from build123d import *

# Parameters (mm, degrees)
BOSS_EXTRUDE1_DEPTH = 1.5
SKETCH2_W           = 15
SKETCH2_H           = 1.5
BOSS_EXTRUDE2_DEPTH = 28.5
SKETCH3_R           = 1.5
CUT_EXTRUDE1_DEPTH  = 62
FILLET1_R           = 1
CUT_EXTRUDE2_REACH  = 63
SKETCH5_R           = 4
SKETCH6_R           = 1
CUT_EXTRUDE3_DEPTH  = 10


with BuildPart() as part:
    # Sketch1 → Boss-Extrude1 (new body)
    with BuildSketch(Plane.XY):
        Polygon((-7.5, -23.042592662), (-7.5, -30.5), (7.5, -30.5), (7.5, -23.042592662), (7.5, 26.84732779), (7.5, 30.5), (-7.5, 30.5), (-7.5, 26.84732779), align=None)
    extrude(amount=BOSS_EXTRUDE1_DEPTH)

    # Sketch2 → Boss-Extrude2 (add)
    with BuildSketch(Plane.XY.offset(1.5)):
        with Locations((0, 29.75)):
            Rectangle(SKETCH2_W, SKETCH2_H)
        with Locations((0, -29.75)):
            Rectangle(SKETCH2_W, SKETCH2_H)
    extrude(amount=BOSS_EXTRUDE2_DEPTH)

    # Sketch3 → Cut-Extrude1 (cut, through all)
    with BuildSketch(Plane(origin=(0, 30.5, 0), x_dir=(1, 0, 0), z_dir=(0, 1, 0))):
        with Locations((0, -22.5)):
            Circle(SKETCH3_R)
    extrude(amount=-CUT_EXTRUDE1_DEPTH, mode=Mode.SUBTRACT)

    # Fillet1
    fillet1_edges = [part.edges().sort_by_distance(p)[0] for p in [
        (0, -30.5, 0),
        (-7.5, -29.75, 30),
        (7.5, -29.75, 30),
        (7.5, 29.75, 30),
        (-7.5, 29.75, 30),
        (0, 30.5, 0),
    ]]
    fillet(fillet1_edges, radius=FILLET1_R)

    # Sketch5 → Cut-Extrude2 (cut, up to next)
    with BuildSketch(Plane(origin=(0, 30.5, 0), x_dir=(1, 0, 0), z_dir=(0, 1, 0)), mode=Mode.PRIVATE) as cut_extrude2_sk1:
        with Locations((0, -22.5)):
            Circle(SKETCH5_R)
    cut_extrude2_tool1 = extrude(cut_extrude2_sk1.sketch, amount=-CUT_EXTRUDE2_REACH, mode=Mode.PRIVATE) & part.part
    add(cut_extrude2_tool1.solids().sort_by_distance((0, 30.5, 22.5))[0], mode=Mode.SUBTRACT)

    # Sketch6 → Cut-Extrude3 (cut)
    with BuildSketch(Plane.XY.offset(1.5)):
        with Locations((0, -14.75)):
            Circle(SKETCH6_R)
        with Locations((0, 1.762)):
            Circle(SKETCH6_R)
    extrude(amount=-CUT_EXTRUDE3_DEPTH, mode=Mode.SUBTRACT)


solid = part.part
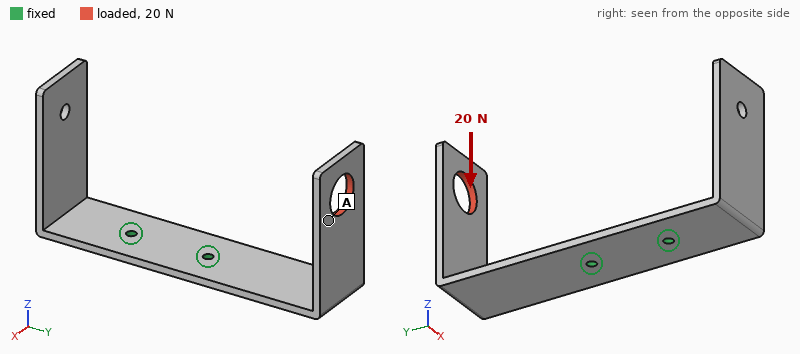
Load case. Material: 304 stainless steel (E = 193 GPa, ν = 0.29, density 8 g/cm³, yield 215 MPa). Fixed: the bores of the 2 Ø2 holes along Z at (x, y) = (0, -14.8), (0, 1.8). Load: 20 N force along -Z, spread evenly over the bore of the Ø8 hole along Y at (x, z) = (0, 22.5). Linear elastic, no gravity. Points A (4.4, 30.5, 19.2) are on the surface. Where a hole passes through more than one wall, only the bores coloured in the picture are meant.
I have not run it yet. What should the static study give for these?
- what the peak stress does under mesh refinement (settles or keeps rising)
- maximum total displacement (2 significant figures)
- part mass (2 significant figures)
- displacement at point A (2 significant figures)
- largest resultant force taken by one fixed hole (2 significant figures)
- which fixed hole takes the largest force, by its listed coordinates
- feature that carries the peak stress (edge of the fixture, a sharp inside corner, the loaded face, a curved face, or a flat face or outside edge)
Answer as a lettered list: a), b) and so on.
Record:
a) keeps rising
b) 0.34 mm
c) 20 g
d) 0.26 mm
e) 28 N
f) (0, 1.8)
g) edge of the fixture
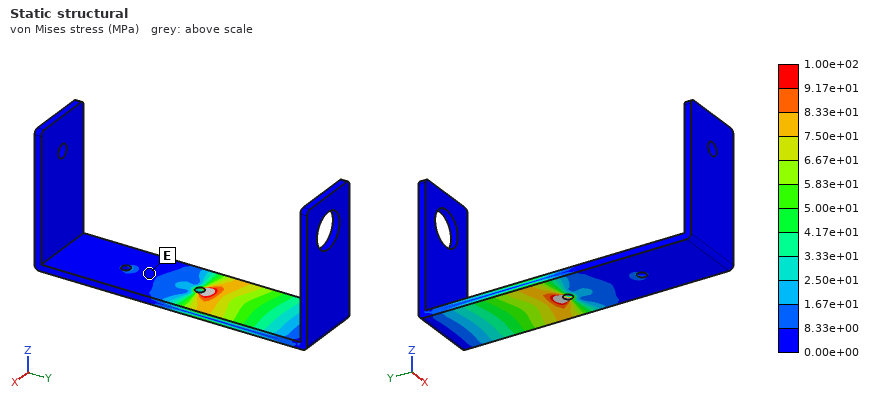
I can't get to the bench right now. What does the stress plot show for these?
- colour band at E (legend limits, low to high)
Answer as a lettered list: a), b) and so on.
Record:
a) 0.00e+00 to 8.33e+00 MPa
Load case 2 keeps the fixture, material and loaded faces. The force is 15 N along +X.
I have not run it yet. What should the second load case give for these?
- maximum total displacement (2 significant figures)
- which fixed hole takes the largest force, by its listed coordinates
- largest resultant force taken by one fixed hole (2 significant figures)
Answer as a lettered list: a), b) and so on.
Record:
a) 0.22 mm
b) (0, 1.8)
c) 37 N
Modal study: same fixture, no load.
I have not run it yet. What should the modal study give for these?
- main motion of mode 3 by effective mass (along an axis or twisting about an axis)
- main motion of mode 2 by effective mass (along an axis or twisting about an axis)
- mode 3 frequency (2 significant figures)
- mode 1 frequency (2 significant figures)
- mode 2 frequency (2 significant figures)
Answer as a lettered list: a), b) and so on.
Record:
a) along X
b) along Y
c) 910 Hz
d) 530 Hz
e) 770 Hz
